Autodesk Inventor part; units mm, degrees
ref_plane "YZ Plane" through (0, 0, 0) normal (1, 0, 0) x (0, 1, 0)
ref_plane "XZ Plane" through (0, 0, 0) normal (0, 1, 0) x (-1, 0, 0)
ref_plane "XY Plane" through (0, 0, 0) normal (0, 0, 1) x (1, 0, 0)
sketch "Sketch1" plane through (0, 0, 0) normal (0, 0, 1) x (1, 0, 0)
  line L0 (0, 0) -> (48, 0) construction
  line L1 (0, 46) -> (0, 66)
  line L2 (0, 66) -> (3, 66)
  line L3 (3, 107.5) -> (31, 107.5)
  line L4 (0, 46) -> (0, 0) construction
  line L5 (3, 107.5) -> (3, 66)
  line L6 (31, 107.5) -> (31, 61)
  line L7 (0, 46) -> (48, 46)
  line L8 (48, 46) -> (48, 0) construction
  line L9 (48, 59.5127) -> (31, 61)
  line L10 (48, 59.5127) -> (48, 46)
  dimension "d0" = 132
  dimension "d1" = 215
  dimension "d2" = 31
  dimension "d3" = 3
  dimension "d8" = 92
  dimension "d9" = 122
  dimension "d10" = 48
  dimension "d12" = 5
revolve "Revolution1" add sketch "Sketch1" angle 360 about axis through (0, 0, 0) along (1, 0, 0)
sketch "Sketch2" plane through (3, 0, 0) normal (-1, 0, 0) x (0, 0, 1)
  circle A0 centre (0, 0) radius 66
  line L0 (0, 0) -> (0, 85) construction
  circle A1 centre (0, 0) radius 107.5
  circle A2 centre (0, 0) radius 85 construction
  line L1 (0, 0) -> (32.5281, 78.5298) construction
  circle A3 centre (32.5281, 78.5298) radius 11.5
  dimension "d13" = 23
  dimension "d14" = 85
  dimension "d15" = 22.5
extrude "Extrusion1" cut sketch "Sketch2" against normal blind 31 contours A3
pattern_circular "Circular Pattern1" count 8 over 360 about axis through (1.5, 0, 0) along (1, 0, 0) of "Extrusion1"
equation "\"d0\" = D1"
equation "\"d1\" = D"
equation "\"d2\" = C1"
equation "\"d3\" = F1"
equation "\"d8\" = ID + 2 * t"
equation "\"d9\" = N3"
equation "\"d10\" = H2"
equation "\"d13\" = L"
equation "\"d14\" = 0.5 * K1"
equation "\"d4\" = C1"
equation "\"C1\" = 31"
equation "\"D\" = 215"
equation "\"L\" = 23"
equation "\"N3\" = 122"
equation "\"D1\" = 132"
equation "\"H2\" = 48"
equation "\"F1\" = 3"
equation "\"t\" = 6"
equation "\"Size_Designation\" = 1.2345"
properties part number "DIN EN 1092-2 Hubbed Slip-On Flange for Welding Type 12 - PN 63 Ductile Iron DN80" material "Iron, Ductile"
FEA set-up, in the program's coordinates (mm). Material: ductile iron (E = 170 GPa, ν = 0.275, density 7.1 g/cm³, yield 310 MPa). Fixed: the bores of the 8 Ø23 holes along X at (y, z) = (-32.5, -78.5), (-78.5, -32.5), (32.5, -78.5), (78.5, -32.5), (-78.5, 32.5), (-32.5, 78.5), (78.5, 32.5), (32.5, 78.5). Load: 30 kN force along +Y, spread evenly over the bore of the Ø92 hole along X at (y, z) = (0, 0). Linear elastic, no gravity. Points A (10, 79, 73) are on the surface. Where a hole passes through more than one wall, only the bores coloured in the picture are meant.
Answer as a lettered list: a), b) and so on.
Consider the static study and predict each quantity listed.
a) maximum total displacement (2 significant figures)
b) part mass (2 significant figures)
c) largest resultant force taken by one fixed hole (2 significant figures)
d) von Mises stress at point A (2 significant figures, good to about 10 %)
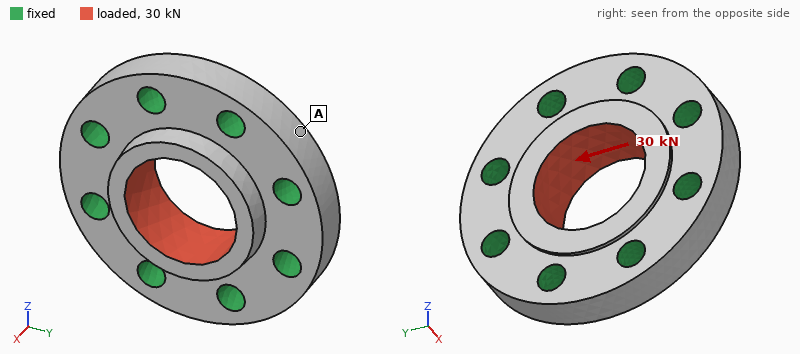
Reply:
a) 2.6 µm
b) 6.0 kg
c) 5.1 kN
d) 0.86 MPa
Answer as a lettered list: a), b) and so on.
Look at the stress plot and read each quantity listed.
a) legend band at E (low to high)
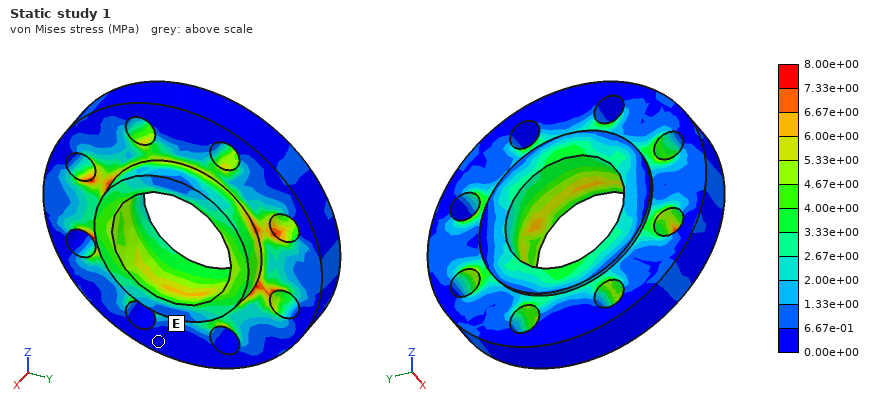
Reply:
a) 0.00e+00 to 6.67e-01 MPa
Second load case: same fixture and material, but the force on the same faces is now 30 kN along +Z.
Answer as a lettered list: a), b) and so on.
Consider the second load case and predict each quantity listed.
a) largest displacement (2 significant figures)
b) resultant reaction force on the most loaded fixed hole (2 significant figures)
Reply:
a) 2.5 µm
b) 5.1 kN
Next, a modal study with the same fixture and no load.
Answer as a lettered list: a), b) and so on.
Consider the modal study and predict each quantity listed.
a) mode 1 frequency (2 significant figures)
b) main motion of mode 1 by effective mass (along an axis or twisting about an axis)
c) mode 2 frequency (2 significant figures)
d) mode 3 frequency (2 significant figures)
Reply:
a) 13 kHz
b) along X
c) 15 kHz
d) 15 kHz
